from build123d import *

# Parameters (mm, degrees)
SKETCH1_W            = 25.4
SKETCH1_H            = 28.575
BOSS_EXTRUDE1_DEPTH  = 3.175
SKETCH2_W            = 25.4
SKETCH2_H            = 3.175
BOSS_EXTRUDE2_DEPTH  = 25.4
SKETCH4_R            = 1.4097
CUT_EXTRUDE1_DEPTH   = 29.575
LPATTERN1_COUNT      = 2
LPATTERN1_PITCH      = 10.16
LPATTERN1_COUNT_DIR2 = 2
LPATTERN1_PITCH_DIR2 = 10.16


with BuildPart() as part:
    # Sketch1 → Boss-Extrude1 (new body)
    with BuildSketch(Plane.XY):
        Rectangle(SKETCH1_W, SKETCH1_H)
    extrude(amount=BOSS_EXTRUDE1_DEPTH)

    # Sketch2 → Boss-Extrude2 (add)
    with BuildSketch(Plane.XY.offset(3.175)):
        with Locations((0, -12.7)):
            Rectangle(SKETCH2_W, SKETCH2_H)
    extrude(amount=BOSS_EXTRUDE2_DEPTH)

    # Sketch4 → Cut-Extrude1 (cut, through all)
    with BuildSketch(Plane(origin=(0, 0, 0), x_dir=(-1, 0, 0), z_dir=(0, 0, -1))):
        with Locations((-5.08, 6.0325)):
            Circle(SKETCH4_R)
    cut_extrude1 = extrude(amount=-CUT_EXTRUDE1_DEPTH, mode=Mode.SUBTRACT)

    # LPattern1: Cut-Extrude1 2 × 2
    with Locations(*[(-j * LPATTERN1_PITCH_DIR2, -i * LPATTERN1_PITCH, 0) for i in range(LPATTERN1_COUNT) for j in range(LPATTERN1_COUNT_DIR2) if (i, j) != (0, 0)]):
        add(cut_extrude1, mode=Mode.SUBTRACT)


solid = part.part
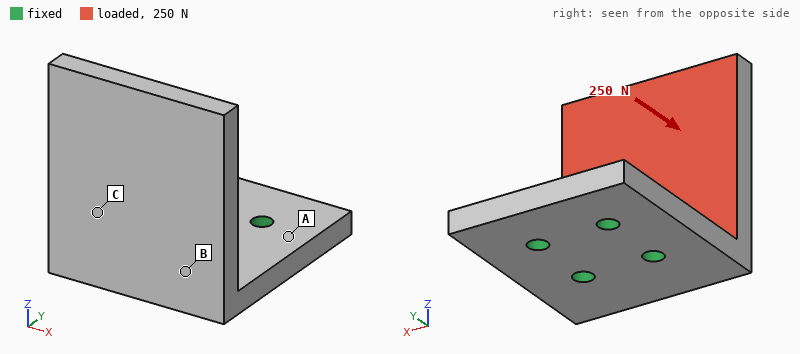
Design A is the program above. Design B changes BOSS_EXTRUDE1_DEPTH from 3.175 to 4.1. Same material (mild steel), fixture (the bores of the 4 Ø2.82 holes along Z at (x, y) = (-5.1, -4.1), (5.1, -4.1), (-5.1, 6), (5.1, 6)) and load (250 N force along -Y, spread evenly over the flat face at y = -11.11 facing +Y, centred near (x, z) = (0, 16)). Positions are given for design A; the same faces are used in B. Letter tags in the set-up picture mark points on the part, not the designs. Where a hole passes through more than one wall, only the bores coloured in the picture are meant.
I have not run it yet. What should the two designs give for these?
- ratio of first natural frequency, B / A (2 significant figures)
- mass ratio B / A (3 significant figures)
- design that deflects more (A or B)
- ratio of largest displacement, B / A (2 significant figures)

1.3
1.13
A
0.67
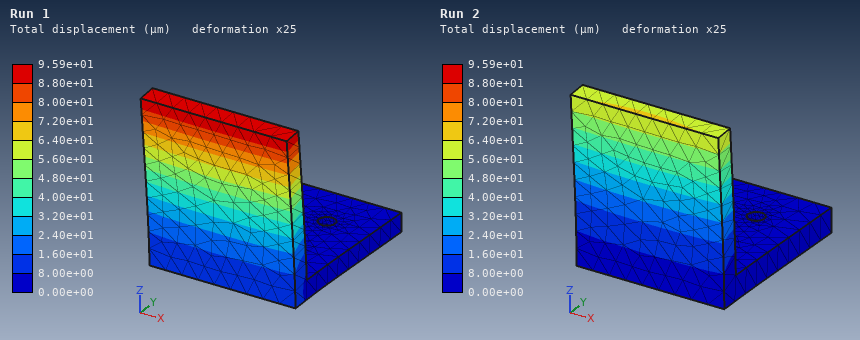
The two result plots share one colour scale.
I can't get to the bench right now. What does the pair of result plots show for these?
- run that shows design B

Run 2
